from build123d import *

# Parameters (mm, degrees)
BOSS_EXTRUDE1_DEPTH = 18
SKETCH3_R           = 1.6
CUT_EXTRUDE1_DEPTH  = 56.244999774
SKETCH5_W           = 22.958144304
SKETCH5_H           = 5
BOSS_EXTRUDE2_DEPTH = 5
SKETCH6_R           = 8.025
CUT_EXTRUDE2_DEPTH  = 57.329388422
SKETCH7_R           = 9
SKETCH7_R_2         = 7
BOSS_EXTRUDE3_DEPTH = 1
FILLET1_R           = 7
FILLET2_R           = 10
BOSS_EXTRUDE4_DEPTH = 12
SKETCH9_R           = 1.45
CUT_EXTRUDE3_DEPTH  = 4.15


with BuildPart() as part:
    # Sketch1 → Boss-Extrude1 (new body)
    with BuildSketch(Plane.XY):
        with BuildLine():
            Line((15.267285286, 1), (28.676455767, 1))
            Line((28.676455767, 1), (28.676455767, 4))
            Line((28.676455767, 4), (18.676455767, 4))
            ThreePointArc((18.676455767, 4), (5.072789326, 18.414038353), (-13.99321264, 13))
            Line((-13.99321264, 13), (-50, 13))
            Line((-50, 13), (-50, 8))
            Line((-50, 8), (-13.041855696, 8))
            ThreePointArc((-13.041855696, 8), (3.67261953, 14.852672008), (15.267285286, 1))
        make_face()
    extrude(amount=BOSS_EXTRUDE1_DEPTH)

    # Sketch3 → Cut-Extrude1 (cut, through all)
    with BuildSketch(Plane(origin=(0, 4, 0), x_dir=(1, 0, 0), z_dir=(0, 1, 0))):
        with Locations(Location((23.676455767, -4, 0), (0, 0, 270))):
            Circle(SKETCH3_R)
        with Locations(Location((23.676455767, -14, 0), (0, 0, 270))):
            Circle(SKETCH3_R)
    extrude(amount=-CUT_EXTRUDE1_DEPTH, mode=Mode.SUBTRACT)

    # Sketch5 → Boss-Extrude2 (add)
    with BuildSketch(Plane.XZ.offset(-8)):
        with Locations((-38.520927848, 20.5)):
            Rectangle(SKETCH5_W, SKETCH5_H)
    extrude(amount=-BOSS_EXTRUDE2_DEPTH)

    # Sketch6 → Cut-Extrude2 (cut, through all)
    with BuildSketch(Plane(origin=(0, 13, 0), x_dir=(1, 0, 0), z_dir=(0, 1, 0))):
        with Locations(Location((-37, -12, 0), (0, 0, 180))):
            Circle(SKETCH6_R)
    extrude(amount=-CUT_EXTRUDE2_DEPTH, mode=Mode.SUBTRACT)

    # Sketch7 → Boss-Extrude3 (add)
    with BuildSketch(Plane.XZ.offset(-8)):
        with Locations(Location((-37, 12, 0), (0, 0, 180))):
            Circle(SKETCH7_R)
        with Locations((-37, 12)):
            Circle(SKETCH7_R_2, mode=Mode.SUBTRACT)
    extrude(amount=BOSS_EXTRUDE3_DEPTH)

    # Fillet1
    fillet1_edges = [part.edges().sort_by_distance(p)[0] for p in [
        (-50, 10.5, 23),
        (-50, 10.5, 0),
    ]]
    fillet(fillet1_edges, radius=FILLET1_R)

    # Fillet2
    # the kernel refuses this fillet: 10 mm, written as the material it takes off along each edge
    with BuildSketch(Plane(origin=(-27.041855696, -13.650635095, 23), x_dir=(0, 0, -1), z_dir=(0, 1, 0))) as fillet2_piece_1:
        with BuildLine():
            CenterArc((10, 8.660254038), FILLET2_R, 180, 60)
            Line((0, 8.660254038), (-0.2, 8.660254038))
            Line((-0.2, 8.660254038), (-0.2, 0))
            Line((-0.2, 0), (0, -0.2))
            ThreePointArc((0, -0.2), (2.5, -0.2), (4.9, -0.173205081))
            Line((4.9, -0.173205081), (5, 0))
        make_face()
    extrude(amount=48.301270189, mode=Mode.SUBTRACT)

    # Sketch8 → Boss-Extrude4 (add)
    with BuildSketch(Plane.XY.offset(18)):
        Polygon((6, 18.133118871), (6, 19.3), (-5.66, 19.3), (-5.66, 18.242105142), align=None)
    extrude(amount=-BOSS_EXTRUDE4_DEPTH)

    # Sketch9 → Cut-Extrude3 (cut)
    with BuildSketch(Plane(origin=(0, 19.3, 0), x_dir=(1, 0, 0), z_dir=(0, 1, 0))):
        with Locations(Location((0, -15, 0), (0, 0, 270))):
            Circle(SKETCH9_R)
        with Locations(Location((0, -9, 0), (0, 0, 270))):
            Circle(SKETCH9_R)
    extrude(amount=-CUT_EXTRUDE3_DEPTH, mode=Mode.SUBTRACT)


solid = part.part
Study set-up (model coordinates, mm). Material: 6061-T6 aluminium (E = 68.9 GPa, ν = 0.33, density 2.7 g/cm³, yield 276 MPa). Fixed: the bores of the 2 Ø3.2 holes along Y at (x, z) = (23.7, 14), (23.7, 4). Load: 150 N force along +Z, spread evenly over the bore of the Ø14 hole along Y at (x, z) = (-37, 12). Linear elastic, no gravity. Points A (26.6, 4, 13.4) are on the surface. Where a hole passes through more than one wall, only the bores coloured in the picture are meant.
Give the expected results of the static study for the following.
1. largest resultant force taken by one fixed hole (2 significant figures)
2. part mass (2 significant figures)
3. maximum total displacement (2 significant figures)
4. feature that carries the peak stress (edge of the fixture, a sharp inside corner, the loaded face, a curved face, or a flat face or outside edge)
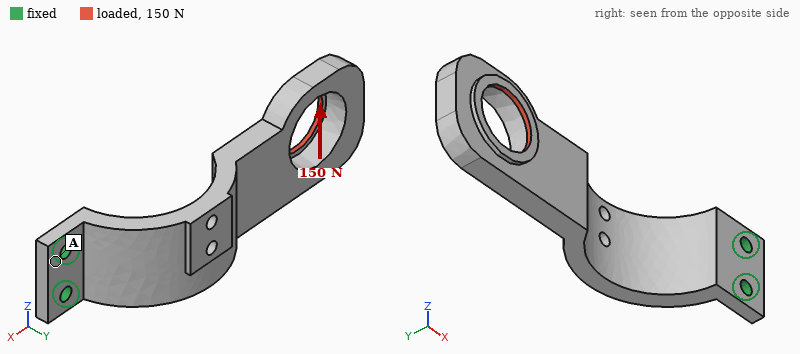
780 N
17 g
0.79 mm
a curved face
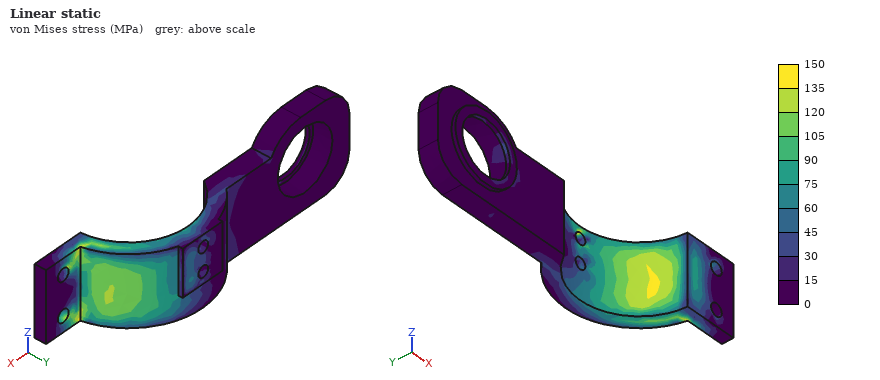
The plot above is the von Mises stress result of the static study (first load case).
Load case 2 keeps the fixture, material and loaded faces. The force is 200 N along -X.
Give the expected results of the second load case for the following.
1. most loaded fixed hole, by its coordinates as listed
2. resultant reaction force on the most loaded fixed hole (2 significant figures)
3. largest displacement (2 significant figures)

(23.7, 14)
150 N
0.32 mm
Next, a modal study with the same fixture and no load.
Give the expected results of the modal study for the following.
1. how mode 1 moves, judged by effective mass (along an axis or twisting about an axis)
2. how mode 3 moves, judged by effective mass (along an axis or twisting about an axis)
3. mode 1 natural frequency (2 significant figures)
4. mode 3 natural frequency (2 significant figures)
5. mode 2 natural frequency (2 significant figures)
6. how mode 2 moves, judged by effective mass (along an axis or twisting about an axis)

along Y
along X
460 Hz
2300 Hz
990 Hz
along Z
